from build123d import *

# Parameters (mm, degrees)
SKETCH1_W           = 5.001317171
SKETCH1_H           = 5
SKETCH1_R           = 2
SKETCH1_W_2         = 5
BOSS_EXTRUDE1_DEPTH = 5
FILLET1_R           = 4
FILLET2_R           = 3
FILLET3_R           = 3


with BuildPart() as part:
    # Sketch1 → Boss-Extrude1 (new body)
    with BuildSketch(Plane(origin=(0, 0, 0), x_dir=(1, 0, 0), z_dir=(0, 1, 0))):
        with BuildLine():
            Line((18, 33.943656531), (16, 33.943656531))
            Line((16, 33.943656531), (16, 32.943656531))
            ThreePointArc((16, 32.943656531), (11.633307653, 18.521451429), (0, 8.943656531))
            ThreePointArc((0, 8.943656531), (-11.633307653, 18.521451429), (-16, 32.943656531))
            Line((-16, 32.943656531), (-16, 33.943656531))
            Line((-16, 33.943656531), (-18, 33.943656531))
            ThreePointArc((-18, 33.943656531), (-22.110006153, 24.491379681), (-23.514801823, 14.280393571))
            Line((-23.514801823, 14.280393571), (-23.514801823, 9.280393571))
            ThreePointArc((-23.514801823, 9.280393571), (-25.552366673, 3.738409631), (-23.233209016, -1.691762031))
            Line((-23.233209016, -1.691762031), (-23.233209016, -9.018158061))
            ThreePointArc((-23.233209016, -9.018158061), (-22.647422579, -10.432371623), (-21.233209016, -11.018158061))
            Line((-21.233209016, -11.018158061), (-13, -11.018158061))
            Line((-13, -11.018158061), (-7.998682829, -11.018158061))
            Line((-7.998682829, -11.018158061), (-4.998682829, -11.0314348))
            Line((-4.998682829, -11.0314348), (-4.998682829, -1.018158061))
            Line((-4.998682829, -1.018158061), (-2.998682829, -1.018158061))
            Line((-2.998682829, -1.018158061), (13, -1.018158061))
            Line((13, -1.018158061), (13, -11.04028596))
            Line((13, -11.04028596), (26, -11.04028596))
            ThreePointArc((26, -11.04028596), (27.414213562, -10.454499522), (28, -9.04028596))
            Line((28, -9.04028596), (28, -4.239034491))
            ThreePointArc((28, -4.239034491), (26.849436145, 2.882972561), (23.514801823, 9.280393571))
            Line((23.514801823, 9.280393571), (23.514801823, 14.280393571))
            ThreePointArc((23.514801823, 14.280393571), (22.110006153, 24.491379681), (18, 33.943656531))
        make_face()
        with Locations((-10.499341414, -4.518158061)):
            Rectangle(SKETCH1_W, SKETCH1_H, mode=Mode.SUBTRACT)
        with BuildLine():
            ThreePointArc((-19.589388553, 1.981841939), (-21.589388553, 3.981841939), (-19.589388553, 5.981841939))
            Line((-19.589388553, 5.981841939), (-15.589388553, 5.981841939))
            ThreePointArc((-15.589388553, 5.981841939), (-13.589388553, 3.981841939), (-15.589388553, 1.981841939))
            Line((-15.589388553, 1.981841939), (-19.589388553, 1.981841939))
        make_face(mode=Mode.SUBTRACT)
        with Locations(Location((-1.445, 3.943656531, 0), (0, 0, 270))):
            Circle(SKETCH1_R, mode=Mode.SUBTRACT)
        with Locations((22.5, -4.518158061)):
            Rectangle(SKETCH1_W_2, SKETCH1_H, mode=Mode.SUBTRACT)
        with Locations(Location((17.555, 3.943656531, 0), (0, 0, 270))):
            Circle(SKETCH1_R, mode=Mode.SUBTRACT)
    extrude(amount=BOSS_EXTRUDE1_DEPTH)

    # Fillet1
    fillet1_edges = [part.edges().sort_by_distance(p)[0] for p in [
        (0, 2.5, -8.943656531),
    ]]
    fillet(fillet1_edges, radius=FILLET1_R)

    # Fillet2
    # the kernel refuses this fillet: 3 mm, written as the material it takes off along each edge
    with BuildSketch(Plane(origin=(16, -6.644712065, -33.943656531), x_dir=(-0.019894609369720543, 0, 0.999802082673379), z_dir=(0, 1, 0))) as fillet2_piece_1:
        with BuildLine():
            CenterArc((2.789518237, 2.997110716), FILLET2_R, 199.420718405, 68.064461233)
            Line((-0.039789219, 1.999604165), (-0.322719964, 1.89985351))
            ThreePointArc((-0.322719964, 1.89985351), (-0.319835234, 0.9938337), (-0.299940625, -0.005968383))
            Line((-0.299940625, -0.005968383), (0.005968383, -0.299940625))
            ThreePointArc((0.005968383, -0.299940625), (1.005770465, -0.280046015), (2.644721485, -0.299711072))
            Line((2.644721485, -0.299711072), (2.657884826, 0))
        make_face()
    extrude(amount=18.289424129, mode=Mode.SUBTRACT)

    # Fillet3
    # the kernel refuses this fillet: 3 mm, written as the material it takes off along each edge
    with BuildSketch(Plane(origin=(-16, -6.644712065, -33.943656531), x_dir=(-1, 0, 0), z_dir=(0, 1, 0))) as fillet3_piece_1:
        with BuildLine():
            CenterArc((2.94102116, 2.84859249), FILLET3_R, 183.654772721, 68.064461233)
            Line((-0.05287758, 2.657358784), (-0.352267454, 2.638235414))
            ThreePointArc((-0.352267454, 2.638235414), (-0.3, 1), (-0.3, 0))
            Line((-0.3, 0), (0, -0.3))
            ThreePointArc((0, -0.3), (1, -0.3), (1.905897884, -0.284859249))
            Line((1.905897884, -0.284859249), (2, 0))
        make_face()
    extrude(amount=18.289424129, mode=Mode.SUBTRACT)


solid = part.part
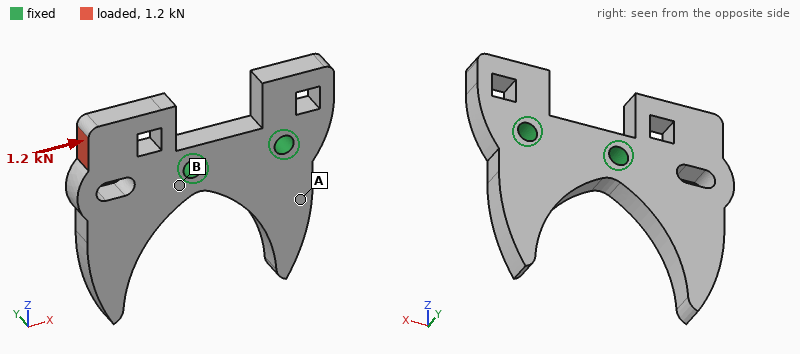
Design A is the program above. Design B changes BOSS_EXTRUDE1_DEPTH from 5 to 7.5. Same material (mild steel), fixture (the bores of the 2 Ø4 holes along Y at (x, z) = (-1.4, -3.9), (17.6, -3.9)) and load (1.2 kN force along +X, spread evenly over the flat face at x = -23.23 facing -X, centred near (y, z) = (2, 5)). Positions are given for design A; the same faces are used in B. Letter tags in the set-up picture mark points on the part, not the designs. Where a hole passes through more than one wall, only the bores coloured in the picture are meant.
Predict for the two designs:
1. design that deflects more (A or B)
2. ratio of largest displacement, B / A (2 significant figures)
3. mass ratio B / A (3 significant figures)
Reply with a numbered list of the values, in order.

1. A
2. 0.66
3. 1.50
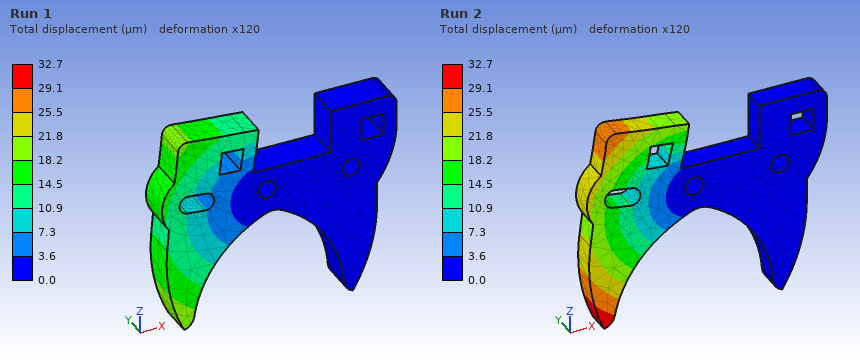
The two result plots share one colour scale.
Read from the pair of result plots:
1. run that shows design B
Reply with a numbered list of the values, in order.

1. Run 1
